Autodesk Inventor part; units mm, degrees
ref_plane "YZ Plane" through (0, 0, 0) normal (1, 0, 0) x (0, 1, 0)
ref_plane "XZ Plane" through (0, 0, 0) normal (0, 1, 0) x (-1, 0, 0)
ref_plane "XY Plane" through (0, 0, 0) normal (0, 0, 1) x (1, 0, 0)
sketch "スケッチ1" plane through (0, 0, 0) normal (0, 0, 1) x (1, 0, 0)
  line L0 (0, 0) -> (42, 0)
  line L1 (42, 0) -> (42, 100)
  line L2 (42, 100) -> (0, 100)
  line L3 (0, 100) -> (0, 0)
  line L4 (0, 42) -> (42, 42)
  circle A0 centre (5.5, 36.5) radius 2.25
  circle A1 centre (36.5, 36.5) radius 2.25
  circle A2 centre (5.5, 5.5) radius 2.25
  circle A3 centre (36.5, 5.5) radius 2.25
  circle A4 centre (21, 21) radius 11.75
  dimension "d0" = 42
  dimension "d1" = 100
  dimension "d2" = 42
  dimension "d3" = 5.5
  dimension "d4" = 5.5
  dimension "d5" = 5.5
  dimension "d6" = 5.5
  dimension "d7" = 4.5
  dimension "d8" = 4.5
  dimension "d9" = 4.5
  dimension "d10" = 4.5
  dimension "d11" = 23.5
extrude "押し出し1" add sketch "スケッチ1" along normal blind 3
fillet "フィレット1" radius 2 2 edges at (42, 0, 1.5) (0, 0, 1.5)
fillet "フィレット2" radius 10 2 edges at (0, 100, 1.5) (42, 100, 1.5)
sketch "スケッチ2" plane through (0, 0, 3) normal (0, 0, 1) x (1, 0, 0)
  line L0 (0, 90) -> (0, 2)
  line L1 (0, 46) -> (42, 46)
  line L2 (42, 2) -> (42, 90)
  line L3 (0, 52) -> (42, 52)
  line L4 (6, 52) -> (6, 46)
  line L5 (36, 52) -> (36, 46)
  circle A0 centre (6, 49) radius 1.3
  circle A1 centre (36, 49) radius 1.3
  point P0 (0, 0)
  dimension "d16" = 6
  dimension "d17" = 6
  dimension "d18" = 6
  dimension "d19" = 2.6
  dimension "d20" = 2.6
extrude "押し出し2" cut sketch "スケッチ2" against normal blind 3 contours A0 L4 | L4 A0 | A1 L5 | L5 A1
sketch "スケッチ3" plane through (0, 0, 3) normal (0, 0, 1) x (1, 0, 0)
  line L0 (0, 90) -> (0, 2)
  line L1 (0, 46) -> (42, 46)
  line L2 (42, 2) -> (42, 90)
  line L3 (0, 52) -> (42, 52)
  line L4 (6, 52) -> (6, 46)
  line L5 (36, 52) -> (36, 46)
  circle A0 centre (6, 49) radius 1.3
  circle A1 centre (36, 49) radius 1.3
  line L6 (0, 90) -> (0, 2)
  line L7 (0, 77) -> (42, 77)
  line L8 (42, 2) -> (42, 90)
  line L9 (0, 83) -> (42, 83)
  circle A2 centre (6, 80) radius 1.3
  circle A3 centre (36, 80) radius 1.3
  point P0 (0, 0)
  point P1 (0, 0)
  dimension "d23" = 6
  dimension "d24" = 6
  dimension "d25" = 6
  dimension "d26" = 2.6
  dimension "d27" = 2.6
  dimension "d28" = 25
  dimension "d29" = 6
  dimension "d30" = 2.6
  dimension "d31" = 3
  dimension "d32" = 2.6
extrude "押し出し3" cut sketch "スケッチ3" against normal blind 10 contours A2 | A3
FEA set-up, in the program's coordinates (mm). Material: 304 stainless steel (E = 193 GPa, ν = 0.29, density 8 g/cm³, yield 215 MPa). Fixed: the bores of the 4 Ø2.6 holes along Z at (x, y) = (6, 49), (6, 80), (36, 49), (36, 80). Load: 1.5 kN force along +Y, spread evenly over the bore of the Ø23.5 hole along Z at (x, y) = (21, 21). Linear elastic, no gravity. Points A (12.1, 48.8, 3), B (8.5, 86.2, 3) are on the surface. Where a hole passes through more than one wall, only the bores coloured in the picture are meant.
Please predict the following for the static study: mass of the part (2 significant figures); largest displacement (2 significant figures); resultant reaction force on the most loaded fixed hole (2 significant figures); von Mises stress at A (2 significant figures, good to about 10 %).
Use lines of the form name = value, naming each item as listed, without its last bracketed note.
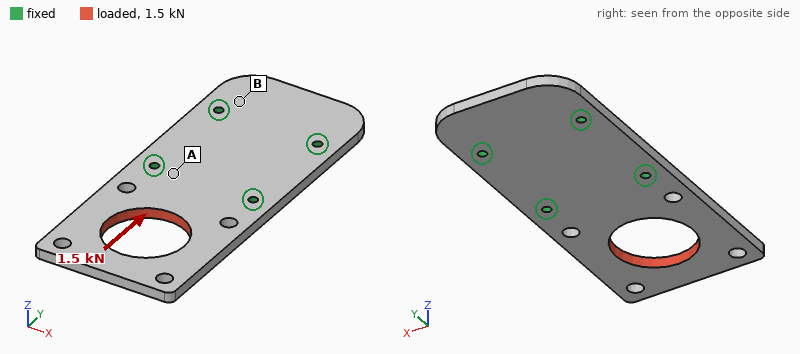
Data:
mass of the part = 87 g
largest displacement = 6.2 µm
resultant reaction force on the most loaded fixed hole = 630 N
von Mises stress at A = 6.1 MPa
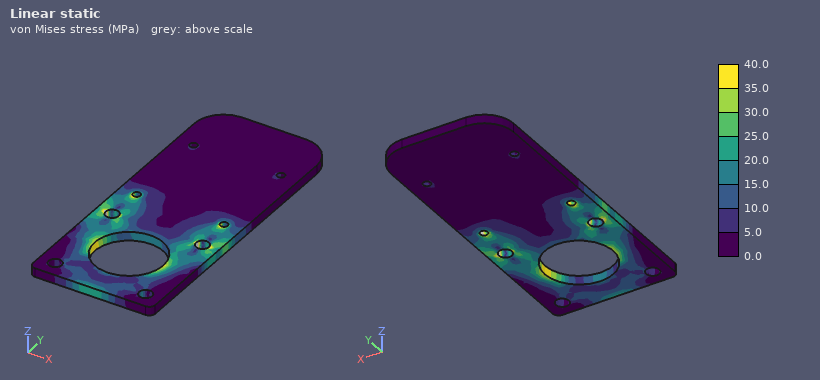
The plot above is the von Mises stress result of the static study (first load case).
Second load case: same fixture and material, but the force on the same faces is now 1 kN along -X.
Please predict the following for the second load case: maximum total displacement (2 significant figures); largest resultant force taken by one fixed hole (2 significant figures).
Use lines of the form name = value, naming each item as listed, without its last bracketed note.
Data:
maximum total displacement = 20 µm
largest resultant force taken by one fixed hole = 940 N
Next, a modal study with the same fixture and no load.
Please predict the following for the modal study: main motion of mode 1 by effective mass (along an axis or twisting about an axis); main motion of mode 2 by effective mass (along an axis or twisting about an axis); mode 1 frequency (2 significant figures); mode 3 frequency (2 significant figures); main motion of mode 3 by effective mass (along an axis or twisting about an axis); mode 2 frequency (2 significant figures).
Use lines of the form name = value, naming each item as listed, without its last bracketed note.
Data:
main motion of mode 1 by effective mass = along Z
main motion of mode 2 by effective mass = twisting about Y
mode 1 frequency = 940 Hz
mode 3 frequency = 5300 Hz
main motion of mode 3 by effective mass = along Z
mode 2 frequency = 2400 Hz
